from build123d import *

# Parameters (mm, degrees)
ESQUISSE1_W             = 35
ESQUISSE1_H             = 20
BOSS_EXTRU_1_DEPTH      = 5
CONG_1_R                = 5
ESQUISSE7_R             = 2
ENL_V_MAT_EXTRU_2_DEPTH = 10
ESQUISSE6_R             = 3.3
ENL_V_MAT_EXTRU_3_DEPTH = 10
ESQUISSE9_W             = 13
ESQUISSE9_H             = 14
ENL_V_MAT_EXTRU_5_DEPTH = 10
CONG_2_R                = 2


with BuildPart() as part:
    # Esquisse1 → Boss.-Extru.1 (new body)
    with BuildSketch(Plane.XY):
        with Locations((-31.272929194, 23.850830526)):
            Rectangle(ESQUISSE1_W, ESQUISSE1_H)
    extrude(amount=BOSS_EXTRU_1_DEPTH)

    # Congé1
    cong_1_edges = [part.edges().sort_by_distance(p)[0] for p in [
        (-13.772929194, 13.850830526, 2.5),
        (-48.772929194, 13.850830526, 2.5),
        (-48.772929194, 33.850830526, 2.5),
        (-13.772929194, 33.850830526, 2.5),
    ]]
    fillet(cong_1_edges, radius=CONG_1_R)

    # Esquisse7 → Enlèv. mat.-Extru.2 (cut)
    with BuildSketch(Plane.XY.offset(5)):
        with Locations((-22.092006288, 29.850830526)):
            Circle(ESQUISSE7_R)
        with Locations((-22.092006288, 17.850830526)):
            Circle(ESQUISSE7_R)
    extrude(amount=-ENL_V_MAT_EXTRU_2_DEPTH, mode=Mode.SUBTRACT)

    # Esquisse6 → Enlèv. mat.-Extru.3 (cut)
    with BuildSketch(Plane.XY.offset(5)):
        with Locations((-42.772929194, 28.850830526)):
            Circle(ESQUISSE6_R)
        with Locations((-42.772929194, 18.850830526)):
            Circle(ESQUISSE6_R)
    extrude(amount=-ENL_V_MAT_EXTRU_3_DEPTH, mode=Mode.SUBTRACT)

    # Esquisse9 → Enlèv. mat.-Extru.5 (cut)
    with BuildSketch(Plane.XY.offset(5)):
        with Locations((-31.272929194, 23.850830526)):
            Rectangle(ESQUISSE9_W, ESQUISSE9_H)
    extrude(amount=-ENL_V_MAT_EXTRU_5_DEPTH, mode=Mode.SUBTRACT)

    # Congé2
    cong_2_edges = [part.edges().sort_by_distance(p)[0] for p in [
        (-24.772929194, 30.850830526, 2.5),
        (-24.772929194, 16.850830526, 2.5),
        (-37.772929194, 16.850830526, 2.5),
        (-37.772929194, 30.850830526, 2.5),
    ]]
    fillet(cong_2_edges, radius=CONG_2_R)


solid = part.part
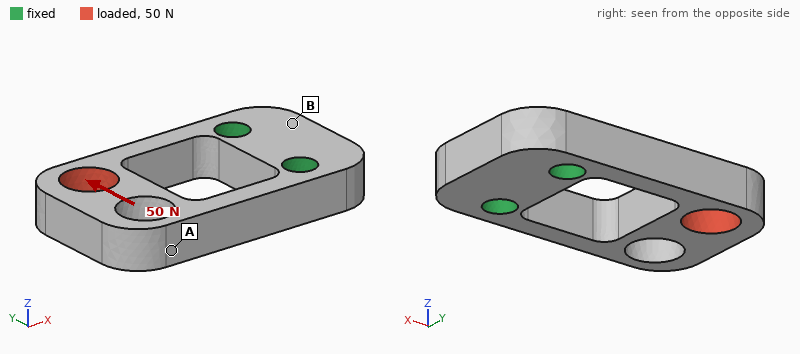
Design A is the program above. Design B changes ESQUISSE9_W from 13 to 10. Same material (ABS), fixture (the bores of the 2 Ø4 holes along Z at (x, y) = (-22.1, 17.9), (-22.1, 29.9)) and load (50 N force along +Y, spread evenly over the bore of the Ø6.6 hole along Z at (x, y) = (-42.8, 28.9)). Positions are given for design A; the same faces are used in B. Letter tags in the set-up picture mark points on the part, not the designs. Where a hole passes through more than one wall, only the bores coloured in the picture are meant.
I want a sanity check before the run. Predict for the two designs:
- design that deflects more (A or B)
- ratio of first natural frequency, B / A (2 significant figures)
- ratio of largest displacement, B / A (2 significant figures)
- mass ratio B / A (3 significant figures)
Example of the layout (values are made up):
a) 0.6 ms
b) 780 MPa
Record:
a) A
b) 1.0
c) 0.58
d) 1.10
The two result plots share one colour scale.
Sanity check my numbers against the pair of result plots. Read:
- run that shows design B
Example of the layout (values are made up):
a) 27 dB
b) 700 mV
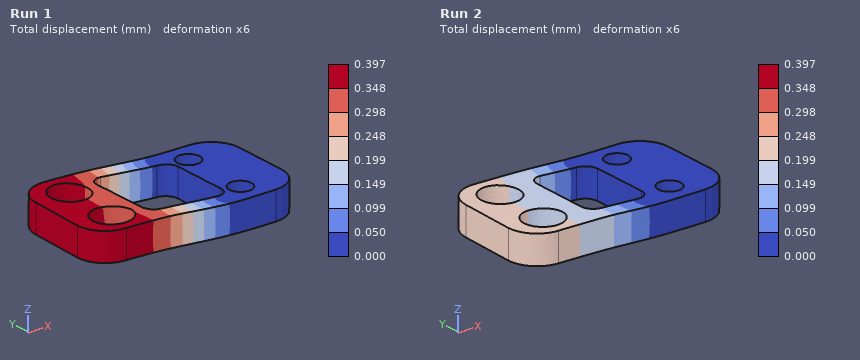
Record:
a) Run 2
